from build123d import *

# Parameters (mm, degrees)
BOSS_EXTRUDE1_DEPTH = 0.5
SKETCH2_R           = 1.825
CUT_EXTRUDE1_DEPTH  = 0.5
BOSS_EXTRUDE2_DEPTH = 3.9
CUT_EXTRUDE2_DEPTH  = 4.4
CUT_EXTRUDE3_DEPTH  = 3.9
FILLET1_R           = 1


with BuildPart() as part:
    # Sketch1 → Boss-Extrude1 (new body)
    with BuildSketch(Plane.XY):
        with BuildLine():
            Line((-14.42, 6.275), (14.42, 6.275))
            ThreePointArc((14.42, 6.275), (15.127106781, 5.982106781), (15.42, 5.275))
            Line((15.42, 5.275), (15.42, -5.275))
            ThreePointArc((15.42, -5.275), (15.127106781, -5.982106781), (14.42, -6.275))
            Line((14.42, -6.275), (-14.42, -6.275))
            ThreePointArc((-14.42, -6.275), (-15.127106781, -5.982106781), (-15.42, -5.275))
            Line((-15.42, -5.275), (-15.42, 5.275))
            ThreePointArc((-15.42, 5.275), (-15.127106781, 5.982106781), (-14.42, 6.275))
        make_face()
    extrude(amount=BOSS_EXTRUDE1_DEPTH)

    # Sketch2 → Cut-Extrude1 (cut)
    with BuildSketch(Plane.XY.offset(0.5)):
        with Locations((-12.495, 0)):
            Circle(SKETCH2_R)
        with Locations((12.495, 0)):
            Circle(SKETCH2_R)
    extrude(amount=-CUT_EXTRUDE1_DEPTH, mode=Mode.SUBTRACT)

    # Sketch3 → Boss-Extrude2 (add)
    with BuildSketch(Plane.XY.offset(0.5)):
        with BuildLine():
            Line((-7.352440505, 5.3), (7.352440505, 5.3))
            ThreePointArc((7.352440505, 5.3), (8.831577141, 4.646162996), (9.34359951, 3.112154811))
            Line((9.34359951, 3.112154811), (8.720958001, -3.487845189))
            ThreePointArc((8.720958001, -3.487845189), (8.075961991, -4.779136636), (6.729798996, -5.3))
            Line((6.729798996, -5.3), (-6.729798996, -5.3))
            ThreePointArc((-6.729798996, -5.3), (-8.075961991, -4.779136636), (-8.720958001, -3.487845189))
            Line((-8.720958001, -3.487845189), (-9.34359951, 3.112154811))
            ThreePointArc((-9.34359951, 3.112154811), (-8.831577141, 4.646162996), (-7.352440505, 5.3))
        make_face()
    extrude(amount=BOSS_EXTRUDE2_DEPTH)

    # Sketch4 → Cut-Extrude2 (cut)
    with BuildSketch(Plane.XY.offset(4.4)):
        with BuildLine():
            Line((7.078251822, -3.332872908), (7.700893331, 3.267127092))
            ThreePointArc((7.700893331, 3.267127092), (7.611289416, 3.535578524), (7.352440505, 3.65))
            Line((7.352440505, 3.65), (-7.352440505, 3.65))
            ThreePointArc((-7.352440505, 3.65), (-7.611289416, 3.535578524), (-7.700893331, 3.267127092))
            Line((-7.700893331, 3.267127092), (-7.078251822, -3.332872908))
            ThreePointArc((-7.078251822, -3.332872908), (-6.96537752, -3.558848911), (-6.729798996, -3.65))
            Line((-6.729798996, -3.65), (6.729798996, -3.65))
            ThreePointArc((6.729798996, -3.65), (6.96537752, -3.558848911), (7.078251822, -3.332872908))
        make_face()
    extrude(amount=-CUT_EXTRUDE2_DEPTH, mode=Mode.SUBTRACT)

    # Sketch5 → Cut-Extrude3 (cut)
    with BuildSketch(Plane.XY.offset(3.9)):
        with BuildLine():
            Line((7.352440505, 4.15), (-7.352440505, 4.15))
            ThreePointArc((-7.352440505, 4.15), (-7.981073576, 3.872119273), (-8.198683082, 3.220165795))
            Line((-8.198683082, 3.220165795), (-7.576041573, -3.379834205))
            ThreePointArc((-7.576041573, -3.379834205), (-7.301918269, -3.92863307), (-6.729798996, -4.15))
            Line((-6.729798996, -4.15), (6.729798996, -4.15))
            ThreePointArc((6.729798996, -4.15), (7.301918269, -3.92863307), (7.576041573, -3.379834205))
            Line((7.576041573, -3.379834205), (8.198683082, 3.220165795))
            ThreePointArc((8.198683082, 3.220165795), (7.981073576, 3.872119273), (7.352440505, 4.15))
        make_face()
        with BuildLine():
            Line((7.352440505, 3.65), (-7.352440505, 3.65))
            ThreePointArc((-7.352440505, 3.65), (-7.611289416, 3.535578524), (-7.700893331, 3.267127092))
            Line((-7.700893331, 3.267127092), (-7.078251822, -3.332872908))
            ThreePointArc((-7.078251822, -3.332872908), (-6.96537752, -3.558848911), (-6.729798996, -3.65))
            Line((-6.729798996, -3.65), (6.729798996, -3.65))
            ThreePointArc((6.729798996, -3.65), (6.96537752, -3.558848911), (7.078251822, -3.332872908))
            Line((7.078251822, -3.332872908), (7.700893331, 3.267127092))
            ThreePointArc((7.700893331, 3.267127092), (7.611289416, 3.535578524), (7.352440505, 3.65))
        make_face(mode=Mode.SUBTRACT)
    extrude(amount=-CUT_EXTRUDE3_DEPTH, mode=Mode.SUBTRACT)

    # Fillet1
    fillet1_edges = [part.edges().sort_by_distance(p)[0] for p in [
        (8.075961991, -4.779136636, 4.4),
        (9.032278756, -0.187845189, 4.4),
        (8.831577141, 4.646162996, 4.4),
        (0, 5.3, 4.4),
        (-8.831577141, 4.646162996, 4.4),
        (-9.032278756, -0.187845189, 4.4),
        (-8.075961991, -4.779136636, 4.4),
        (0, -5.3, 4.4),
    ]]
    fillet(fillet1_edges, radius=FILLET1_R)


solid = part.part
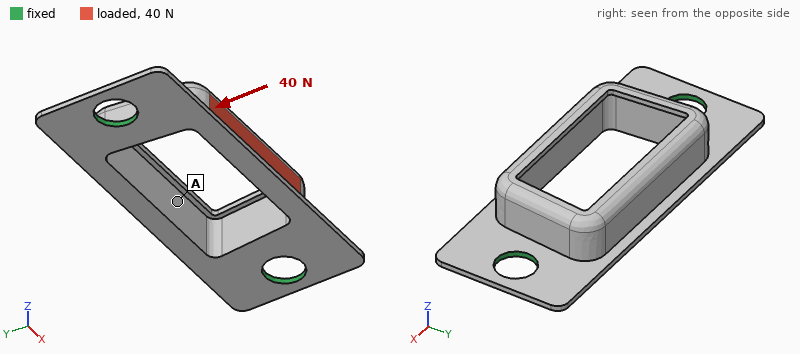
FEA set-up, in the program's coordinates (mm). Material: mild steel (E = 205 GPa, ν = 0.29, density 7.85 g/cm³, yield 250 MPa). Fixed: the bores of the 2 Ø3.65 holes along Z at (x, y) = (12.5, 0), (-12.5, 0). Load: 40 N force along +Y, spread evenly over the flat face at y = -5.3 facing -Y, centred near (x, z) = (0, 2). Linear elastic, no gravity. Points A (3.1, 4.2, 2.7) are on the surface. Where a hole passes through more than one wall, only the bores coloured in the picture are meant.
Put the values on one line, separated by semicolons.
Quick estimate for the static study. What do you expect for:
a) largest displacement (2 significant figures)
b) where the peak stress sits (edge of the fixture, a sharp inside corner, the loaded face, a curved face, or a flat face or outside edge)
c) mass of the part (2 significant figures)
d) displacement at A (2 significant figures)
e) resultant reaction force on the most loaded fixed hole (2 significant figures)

8.5 µm; a curved face; 2.7 g; 3.6 µm; 22 N
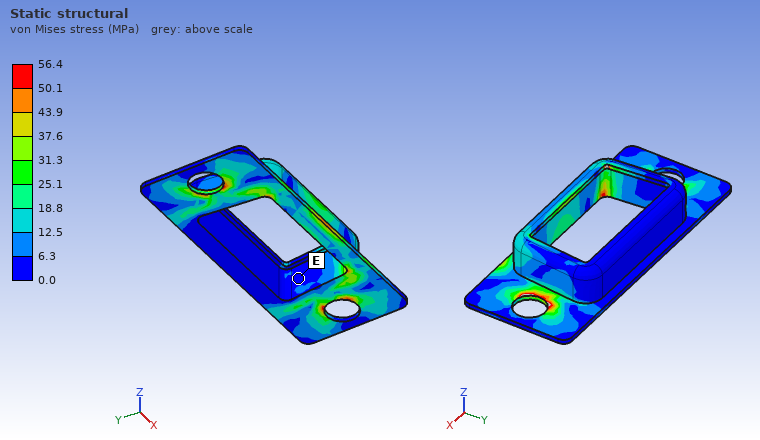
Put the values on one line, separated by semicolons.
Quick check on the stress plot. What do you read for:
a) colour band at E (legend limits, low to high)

0.0 to 6.3 MPa
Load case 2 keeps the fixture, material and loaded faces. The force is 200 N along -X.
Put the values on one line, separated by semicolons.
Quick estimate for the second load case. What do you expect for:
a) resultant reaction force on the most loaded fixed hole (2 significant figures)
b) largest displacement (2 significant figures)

100 N; 5.6 µm
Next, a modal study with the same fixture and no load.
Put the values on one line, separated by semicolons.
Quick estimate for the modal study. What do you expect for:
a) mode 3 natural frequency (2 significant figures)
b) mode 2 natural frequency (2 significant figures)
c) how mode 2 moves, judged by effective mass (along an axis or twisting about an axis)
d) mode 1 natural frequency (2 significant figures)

17 kHz; 15 kHz; along Z; 6500 Hz
